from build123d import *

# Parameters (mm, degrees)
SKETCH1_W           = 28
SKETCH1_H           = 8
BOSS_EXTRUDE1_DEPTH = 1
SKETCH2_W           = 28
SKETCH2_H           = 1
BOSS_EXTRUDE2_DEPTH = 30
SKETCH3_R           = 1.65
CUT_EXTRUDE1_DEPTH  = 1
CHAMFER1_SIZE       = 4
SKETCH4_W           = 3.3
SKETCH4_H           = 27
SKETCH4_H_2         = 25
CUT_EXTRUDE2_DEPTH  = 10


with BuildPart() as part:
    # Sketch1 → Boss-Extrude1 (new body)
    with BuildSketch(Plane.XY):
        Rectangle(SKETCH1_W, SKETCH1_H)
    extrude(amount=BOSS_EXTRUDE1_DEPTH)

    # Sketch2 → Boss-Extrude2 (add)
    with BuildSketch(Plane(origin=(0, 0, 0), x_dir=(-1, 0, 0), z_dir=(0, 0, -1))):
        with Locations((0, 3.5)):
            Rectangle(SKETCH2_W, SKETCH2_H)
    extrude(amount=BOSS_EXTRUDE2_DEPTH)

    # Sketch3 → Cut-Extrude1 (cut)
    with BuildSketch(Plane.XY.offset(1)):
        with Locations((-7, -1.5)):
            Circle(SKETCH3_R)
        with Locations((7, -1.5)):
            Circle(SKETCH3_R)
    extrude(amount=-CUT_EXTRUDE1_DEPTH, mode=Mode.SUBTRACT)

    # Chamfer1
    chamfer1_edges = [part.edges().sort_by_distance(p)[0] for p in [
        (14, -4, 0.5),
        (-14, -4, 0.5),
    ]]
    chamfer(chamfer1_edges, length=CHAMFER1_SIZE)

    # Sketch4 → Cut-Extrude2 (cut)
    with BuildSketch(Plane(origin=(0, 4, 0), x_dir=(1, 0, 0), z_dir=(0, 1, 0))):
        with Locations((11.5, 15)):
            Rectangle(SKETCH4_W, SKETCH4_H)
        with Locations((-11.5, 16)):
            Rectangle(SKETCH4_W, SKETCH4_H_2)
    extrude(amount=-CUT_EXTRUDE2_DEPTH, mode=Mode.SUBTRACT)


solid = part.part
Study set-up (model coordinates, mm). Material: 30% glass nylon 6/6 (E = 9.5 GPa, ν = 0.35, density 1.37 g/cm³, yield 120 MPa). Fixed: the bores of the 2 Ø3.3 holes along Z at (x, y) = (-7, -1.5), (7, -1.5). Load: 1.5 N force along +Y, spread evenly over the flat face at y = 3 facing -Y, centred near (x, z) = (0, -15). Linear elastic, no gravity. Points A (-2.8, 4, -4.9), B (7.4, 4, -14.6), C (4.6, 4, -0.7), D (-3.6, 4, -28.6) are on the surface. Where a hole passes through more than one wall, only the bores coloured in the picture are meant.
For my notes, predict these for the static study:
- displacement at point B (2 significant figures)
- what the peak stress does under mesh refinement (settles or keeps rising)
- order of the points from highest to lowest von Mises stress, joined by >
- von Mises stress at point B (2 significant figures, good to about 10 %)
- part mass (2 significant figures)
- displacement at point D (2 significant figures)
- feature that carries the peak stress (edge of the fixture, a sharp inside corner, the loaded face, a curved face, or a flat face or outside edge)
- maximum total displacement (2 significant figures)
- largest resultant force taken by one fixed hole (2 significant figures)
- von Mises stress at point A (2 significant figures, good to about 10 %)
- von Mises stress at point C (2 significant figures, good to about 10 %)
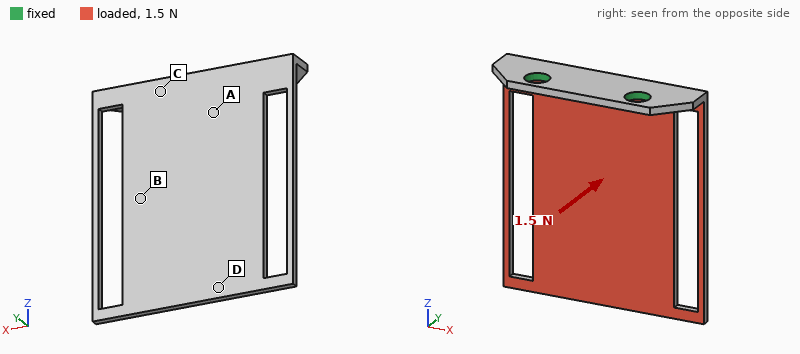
0.16 mm
keeps rising
C > A > B > D
1.7 MPa
1.2 g
0.38 mm
edge of the fixture
0.41 mm
0.81 N
3.7 MPa
4.9 MPa
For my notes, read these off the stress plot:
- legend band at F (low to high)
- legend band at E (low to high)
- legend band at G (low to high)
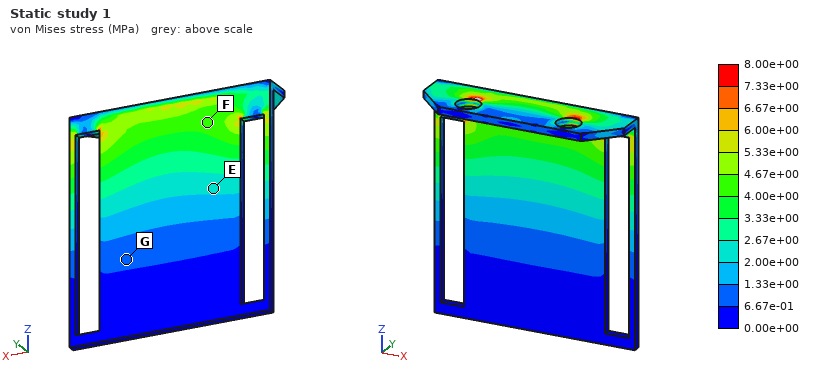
4.00e+00 to 4.67e+00 MPa
2.00e+00 to 2.67e+00 MPa
6.67e-01 to 1.33e+00 MPa
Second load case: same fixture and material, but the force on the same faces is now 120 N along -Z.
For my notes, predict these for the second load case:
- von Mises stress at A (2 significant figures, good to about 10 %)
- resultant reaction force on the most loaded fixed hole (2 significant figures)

8.8 MPa
61 N
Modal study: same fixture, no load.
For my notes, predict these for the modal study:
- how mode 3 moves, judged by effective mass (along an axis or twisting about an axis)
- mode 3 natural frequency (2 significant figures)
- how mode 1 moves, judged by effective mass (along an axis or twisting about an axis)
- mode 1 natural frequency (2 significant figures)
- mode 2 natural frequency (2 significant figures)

along X
2100 Hz
along Y
390 Hz
1200 Hz
